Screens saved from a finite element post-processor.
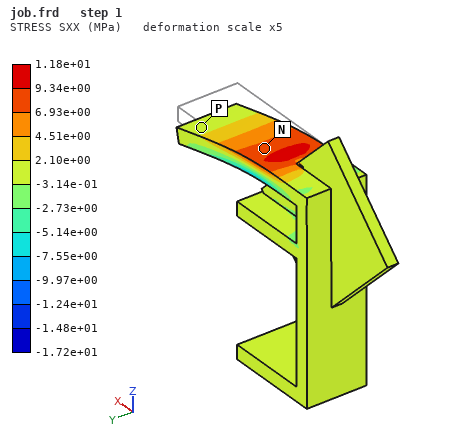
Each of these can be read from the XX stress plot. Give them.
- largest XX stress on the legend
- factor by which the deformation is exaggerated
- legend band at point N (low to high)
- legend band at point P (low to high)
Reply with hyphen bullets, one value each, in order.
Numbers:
- 1.18e+01 MPa
- 5
- 6.93e+00 to 9.34e+00 MPa
- -3.14e-01 to 2.10e+00 MPa
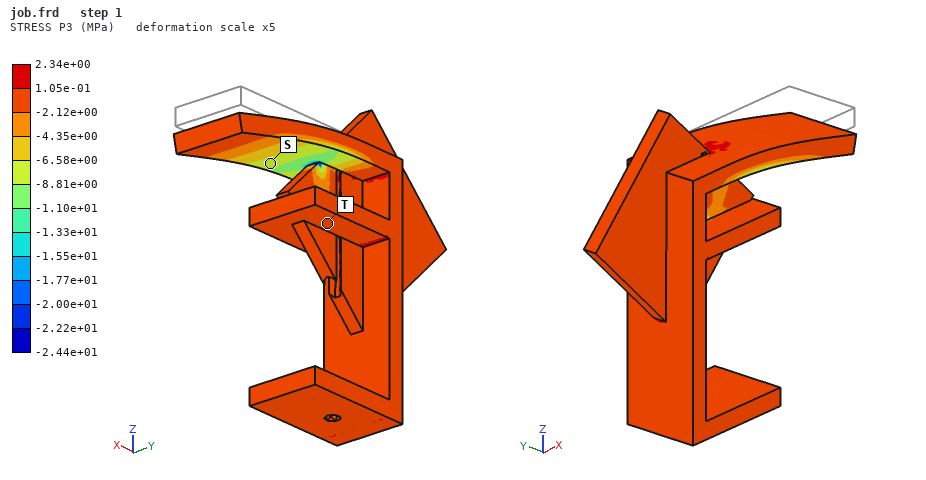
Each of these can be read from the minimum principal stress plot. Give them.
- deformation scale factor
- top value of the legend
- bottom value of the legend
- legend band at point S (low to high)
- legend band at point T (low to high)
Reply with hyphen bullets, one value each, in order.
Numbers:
- 5
- 2.34e+00 MPa
- -2.44e+01 MPa
- -8.81e+00 to -6.58e+00 MPa
- -2.12e+00 to 1.05e-01 MPa
